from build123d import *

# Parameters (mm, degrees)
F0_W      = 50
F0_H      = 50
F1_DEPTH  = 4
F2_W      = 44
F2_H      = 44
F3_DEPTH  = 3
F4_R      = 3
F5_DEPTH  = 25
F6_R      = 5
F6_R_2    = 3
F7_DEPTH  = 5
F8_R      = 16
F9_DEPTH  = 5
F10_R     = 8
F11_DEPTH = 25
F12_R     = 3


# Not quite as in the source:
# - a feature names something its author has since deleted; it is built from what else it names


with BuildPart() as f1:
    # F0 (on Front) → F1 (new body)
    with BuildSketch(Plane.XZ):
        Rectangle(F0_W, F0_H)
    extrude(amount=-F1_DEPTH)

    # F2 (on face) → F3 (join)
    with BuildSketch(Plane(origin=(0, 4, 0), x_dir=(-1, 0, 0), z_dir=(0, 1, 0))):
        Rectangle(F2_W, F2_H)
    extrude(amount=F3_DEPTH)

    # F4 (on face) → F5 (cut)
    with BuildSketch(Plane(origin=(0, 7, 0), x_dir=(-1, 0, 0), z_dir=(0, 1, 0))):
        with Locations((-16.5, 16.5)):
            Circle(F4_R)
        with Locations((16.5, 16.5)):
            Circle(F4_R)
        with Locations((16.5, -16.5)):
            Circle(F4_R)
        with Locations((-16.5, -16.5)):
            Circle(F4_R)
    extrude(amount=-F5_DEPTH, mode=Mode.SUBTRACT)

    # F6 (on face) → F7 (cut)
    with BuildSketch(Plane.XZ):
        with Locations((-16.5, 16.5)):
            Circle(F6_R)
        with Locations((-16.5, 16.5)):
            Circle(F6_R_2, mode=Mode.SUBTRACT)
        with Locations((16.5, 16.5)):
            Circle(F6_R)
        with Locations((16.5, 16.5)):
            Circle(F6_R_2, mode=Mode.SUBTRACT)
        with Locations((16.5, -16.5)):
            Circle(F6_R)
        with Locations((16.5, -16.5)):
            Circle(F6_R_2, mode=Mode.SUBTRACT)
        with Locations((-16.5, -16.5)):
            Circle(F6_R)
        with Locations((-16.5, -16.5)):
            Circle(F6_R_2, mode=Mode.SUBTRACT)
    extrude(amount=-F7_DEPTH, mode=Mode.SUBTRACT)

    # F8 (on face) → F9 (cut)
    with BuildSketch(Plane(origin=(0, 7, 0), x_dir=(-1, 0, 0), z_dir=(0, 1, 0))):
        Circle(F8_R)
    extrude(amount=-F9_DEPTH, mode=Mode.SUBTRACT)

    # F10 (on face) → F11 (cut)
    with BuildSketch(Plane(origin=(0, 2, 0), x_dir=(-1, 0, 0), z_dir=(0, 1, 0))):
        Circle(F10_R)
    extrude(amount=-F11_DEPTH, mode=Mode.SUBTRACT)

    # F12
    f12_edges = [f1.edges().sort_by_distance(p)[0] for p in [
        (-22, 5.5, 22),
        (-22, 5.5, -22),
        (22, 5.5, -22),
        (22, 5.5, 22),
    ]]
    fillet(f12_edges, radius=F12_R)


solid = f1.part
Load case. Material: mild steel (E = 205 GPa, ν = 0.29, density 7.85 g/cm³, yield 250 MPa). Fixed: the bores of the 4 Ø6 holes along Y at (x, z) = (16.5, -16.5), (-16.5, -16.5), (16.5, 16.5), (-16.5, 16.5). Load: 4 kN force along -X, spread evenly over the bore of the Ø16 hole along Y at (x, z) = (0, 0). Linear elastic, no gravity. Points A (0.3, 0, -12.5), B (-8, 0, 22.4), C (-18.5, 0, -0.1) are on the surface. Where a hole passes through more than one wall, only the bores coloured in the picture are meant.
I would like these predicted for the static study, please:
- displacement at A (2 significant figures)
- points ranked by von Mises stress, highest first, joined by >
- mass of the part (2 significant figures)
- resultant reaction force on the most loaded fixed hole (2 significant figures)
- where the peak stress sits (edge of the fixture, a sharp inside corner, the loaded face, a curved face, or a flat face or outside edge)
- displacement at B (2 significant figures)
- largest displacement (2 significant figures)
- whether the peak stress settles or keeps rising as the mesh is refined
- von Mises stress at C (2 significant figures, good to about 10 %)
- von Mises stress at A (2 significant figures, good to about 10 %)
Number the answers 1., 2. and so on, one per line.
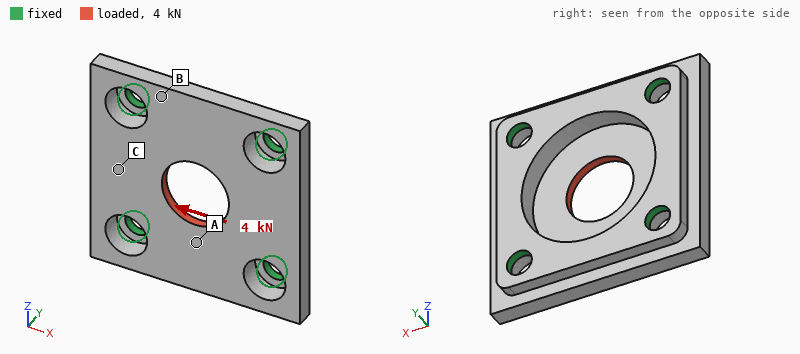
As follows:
1. 2.7 µm
2. A > C > B
3. 75 g
4. 1.0 kN
5. edge of the fixture
6. 1.3 µm
7. 7.2 µm
8. keeps rising
9. 17 MPa
10. 30 MPa
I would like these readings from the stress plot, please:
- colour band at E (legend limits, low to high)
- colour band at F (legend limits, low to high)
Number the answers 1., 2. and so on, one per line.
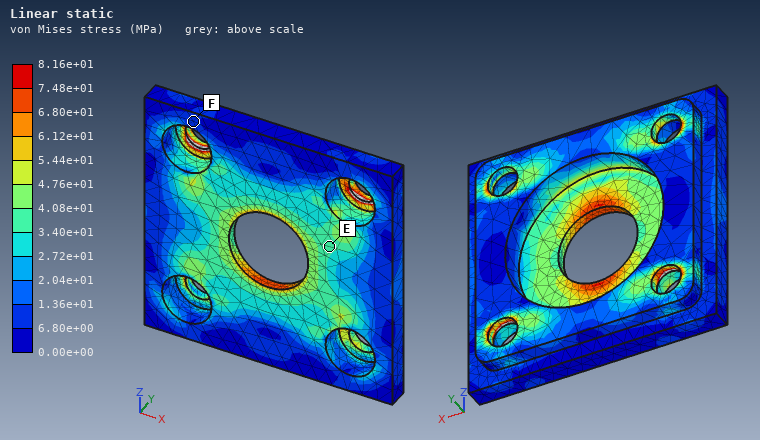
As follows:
1. 3.40e+01 to 4.08e+01 MPa
2. 6.80e+00 to 1.36e+01 MPa
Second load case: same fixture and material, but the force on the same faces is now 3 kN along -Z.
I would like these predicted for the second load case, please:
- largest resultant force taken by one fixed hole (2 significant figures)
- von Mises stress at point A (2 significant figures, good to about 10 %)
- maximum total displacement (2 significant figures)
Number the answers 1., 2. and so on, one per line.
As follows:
1. 770 N
2. 23 MPa
3. 5.4 µm
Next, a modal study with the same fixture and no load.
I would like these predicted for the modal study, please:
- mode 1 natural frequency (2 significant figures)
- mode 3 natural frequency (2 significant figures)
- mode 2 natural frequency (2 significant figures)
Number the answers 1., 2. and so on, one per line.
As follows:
1. 20 kHz
2. 21 kHz
3. 20 kHz
